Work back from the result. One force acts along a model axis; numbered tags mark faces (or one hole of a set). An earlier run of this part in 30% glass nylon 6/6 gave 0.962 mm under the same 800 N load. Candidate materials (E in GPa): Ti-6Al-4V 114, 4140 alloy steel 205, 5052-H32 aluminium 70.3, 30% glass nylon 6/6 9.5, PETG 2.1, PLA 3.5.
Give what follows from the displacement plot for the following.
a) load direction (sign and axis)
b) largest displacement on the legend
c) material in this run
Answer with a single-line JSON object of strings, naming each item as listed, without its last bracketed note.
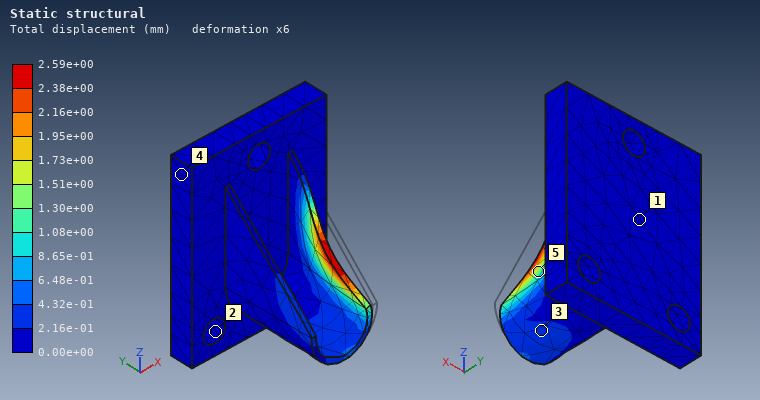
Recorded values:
{"load direction": "-X", "largest displacement on the legend": "2.59e+00 mm", "material in this run": "PLA"}
